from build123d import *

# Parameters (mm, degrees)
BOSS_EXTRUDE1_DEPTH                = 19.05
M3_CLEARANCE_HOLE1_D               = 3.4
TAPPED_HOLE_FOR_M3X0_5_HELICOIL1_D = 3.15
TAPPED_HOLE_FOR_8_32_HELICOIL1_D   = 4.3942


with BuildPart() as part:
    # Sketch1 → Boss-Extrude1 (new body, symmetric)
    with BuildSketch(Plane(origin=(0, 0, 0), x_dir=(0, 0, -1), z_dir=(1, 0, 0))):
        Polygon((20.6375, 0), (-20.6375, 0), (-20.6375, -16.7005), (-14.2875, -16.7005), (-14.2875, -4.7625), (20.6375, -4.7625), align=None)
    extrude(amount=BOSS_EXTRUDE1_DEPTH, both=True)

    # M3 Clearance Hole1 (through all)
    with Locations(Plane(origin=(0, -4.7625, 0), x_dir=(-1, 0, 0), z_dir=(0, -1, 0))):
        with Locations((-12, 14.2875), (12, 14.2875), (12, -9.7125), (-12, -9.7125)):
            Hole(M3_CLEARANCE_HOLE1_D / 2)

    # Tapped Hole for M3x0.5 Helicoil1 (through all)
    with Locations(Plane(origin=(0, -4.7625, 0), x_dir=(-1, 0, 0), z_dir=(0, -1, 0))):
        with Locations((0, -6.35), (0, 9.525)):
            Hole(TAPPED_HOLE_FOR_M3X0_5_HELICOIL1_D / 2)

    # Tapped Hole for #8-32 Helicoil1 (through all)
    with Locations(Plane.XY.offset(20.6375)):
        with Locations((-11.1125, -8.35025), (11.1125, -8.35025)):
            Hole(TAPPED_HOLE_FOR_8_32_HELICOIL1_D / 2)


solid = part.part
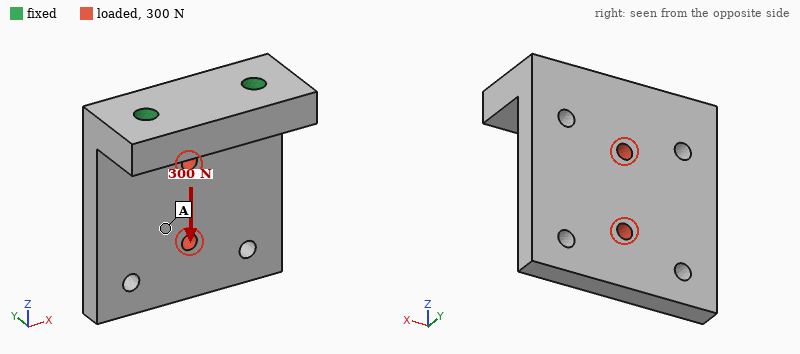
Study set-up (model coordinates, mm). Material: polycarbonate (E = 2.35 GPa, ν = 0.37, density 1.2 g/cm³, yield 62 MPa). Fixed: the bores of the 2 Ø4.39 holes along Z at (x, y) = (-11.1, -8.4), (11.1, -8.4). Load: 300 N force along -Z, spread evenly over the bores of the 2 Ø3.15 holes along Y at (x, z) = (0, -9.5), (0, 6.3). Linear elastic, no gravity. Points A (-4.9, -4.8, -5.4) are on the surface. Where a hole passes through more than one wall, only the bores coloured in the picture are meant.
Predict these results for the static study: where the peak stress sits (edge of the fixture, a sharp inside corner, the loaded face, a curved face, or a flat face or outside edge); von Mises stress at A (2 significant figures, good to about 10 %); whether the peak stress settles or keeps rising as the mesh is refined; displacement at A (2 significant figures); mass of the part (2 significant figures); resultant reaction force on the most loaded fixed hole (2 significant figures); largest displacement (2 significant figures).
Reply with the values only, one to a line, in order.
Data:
edge of the fixture
1.6 MPa
keeps rising
0.094 mm
12 g
150 N
0.16 mm
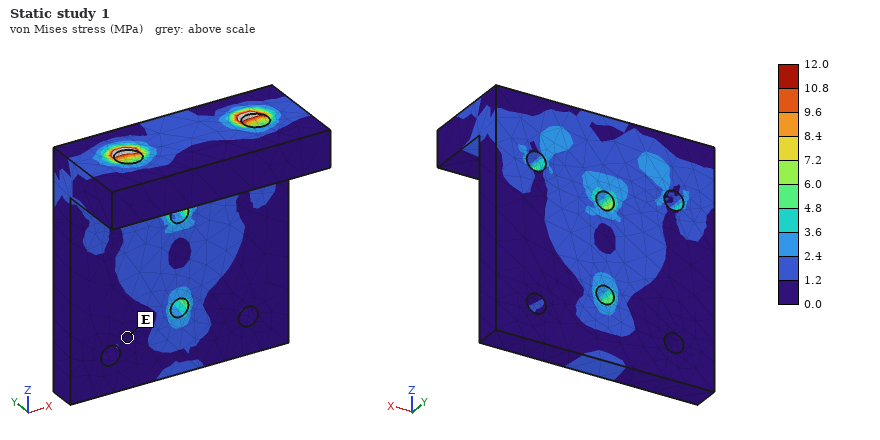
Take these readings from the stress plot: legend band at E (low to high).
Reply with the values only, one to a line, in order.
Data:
0.0 to 1.2 MPa
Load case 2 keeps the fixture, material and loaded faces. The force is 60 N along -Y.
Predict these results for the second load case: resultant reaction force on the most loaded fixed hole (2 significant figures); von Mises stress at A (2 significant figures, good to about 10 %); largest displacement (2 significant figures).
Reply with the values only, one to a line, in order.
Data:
31 N
1.4 MPa
0.57 mm
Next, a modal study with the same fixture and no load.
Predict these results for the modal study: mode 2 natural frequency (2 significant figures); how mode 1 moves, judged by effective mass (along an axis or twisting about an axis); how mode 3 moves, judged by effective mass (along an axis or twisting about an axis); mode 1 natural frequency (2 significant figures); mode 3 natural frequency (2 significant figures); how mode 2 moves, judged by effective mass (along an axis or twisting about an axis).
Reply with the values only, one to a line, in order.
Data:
1700 Hz
along Y
along X
710 Hz
2600 Hz
twisting about Z
